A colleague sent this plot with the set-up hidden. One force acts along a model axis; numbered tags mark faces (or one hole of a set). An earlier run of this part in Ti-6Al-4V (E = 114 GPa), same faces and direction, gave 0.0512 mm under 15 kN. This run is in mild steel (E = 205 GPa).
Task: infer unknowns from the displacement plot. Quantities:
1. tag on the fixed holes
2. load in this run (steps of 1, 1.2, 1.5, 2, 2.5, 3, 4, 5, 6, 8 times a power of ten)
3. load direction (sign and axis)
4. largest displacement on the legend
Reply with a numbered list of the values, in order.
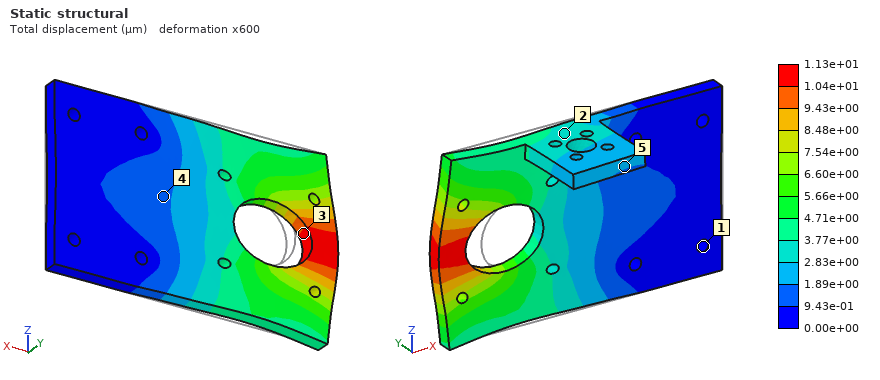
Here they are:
1. 1
2. 6 kN
3. -X
4. 1.13e+01 µm
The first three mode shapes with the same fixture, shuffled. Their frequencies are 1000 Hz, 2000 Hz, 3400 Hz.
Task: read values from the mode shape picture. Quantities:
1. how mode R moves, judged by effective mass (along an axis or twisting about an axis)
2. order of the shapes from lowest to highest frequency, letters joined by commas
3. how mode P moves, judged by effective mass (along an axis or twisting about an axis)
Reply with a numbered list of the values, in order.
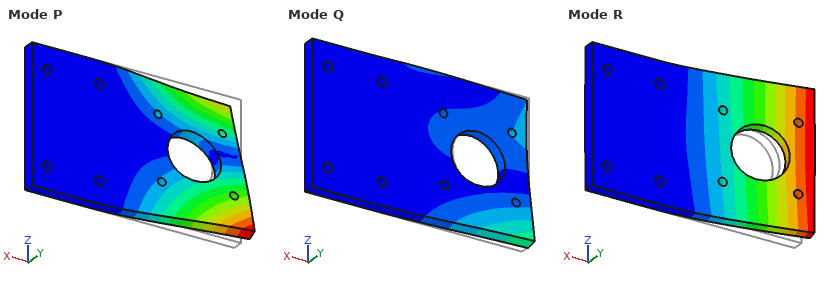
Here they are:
1. along Y
2. R, P, Q
3. twisting about X
